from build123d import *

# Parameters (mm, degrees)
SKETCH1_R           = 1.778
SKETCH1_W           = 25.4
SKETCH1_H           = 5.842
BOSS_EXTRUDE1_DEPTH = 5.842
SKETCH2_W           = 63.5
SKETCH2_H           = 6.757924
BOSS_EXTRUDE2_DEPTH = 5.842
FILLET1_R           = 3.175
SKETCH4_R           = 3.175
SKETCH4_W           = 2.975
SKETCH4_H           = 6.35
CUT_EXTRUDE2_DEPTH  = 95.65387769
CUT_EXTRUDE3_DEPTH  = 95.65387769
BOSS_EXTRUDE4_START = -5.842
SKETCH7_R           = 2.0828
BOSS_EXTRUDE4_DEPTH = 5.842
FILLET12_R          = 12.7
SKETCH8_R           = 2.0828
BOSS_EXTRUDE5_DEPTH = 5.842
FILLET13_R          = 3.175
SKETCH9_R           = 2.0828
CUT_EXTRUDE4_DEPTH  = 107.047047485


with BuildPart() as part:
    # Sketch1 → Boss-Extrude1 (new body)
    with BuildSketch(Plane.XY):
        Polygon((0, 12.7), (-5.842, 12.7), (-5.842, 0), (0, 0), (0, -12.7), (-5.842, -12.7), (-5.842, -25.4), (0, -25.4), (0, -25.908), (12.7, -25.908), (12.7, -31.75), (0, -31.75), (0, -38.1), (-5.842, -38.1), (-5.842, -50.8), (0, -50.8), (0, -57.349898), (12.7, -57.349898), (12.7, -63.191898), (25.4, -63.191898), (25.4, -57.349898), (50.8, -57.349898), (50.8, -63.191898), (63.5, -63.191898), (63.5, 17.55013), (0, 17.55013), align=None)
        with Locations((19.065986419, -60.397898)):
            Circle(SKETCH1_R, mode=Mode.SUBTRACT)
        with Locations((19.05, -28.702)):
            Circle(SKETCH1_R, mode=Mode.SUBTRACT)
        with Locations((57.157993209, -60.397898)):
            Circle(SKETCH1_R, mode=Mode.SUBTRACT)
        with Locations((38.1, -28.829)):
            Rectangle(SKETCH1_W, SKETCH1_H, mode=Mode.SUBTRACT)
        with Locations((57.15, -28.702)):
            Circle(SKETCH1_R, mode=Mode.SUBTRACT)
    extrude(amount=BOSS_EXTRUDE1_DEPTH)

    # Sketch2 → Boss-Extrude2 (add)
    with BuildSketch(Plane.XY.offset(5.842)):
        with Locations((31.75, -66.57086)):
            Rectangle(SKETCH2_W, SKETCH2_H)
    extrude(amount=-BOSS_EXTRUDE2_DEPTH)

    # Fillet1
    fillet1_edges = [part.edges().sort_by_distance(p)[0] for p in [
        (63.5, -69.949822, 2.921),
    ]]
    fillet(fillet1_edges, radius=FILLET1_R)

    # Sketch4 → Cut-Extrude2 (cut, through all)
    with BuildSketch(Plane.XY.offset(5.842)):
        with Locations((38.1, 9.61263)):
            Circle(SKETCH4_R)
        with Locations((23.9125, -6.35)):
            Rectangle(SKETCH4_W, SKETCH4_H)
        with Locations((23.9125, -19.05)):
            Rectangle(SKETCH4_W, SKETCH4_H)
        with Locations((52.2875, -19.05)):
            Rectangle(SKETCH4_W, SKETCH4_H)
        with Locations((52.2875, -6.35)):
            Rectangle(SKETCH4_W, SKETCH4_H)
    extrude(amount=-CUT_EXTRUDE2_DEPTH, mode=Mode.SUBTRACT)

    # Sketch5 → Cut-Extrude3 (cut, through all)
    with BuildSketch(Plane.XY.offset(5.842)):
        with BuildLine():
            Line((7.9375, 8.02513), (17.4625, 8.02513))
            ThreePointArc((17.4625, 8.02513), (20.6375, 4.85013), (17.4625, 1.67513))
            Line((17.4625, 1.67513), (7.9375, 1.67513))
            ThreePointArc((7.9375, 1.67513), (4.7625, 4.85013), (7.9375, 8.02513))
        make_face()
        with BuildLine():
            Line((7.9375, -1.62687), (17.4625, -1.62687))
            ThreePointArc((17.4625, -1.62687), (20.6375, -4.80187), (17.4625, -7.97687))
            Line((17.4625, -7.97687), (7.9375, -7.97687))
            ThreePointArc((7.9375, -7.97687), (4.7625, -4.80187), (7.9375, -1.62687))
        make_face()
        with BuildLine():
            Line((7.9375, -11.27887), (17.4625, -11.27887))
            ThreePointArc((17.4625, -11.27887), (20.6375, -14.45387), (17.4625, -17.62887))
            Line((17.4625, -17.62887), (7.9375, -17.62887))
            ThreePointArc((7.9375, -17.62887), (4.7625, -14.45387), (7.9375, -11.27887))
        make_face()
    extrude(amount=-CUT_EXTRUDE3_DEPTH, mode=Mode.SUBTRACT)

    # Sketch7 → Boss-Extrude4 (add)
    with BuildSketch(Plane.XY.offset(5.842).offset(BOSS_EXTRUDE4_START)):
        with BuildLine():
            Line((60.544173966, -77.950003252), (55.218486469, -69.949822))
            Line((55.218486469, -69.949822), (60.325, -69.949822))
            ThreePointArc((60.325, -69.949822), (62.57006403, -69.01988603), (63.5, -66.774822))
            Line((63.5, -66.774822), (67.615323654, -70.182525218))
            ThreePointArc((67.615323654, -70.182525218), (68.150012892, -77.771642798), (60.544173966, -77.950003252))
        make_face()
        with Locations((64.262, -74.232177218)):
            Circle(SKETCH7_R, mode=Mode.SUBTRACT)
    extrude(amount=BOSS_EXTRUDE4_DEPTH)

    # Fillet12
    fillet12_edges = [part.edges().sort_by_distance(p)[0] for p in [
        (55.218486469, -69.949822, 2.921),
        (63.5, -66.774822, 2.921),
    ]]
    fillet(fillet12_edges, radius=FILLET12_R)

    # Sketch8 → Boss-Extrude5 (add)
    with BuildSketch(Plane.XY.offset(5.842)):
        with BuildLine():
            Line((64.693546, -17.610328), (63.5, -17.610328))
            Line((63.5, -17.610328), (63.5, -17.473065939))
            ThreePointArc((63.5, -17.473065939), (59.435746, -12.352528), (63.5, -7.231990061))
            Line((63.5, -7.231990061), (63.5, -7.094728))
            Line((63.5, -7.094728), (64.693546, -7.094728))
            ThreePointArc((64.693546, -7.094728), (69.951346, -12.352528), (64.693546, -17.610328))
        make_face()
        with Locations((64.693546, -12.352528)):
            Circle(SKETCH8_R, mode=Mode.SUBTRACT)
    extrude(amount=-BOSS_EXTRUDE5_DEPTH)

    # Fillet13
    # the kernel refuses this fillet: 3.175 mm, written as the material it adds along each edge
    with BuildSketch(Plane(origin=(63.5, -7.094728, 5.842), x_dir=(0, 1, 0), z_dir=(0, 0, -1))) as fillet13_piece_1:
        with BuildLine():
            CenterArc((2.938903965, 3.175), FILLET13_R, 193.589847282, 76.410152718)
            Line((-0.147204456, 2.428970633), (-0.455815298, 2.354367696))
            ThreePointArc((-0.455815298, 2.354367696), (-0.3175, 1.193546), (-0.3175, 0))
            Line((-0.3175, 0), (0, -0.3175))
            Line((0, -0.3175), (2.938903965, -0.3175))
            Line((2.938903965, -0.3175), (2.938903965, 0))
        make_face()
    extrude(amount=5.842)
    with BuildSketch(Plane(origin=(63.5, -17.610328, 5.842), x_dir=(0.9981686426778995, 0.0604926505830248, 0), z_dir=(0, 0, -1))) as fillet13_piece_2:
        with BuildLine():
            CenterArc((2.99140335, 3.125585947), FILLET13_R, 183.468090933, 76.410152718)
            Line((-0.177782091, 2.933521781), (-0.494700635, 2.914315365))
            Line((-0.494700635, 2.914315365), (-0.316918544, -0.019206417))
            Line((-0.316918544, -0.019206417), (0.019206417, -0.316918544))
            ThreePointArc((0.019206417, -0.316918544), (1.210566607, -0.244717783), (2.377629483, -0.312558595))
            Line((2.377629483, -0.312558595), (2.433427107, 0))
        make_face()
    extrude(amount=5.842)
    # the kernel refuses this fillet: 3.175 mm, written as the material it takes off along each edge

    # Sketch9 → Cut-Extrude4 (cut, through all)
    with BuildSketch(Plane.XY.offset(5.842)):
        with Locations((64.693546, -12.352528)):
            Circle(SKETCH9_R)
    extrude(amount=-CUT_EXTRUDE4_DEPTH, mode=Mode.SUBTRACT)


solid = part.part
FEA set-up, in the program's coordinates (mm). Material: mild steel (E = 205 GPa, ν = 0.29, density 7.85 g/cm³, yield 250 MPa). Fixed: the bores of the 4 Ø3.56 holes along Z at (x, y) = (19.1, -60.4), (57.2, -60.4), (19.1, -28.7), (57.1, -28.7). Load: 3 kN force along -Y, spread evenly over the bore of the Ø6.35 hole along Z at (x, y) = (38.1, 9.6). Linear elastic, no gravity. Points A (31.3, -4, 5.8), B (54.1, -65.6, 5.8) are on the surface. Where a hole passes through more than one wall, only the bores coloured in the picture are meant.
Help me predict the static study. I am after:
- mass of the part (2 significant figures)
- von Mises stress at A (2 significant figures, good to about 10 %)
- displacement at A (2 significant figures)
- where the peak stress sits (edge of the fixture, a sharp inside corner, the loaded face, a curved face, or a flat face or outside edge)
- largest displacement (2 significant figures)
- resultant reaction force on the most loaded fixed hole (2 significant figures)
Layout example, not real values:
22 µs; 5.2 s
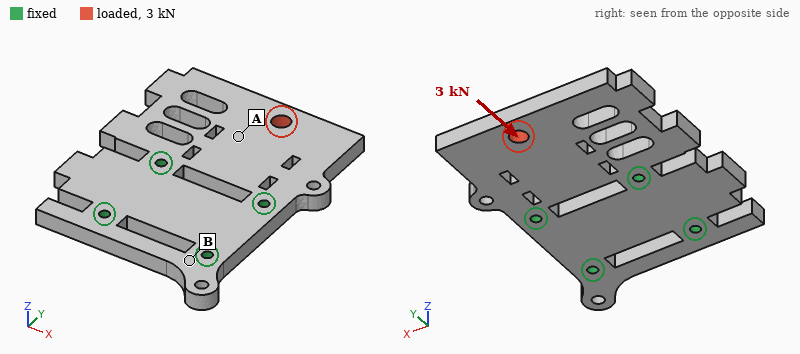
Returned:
230 g; 21 MPa; 3.8 µm; a curved face; 6.4 µm; 1.5 kN
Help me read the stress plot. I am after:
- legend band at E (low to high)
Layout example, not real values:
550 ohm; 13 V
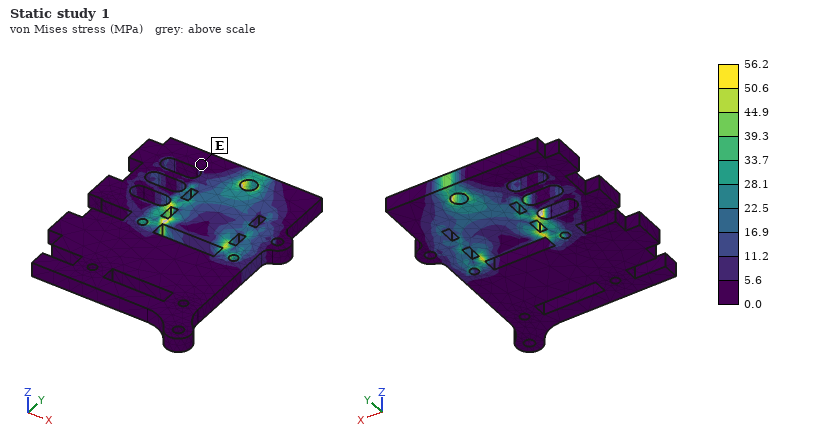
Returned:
0.0 to 5.6 MPa
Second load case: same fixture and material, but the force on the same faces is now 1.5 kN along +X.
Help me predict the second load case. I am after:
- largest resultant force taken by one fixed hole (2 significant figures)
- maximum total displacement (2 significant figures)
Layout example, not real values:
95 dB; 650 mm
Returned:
1.5 kN; 10 µm
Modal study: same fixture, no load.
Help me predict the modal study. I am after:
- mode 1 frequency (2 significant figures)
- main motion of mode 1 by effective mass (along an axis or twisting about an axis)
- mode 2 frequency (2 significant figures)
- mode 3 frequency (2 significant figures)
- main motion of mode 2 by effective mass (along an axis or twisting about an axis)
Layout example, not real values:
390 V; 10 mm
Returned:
1500 Hz; along Z; 3100 Hz; 6700 Hz; twisting about Y
